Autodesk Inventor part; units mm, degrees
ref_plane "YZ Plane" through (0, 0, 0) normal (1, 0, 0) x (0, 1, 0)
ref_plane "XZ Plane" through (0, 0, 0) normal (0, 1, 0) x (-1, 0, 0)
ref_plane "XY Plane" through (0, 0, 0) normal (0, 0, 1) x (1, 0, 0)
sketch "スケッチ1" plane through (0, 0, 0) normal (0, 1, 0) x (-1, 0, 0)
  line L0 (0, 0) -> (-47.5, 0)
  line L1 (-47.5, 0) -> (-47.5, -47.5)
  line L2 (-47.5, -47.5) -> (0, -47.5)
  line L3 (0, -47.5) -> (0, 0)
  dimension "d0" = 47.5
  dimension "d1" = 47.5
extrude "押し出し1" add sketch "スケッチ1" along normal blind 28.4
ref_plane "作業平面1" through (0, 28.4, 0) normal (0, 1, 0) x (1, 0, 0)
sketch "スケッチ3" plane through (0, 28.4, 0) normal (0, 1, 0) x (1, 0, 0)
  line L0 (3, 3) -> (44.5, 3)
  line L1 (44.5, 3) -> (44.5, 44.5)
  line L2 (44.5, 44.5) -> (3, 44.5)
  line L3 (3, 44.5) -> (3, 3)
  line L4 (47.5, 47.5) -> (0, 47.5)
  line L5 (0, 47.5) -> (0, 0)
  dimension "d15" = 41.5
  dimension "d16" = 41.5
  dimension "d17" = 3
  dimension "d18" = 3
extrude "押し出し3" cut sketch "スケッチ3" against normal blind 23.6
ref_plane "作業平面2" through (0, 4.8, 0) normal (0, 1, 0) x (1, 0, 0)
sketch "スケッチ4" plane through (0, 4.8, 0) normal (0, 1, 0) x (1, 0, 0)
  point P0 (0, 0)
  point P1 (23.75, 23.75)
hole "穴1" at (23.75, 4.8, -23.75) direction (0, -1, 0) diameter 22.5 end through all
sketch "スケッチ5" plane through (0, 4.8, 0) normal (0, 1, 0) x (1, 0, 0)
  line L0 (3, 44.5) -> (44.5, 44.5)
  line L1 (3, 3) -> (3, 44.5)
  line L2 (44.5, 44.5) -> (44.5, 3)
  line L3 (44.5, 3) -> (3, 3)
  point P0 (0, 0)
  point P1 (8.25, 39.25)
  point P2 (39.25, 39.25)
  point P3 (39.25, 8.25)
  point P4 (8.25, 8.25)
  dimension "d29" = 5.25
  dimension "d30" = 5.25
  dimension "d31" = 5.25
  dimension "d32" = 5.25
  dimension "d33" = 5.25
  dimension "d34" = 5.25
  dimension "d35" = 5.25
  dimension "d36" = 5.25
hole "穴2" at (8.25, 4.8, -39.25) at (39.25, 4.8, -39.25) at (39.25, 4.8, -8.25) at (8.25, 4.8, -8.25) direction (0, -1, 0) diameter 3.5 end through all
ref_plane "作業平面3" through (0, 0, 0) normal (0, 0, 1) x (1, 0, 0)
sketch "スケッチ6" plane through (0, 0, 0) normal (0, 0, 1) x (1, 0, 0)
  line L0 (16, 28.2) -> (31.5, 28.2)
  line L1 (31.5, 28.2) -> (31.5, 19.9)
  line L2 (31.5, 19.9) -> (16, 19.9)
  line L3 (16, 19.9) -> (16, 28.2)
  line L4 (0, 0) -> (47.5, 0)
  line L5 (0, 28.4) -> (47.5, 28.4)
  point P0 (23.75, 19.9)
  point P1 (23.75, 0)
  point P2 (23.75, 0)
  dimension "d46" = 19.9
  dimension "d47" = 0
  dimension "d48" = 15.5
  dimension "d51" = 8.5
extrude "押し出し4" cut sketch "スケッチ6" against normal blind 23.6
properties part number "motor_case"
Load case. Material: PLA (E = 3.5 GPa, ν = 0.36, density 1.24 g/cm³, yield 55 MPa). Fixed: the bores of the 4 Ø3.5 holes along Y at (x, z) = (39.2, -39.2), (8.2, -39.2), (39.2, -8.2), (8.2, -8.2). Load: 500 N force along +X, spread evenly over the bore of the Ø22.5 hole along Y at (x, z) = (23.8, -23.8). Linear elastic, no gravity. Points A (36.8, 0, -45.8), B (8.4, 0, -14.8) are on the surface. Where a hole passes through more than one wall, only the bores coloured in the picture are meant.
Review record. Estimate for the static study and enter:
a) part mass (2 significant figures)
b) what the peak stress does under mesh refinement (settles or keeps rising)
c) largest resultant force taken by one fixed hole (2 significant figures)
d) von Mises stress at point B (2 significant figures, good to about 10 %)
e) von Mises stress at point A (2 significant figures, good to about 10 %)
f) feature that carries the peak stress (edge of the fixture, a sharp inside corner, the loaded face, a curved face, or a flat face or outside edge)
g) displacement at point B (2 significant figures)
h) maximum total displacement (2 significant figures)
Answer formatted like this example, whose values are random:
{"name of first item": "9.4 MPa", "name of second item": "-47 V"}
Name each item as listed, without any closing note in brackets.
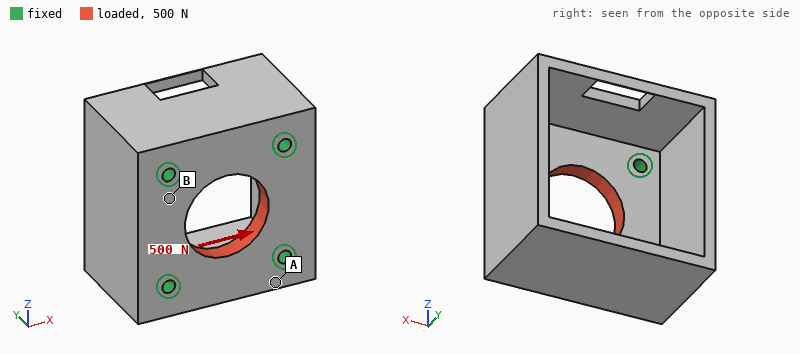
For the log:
{"part mass": "26 g", "what the peak stress does under mesh refinement": "keeps rising", "largest resultant force taken by one fixed hole": "130 N", "von Mises stress at point B": "1.6 MPa", "von Mises stress at point A": "0.45 MPa", "feature that carries the peak stress": "edge of the fixture", "displacement at point B": "7.1 µm", "maximum total displacement": "14 µm"}
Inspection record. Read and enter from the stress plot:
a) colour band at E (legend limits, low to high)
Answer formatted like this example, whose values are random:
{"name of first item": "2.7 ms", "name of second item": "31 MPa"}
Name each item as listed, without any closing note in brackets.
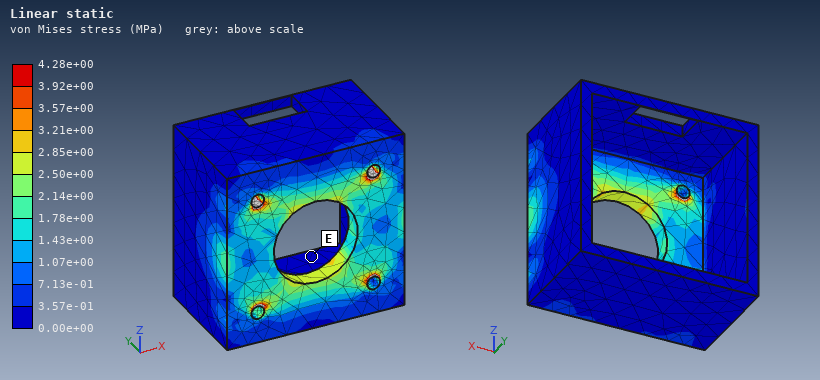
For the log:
{"colour band at E": "0.00e+00 to 3.57e-01 MPa"}
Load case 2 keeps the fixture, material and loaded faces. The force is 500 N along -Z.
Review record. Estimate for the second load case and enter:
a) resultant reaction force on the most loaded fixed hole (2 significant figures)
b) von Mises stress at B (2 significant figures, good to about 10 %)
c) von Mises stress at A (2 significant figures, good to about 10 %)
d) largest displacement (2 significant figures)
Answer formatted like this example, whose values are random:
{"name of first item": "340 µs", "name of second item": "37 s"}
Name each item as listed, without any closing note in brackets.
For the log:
{"resultant reaction force on the most loaded fixed hole": "130 N", "von Mises stress at B": "1.8 MPa", "von Mises stress at A": "0.91 MPa", "largest displacement": "15 µm"}
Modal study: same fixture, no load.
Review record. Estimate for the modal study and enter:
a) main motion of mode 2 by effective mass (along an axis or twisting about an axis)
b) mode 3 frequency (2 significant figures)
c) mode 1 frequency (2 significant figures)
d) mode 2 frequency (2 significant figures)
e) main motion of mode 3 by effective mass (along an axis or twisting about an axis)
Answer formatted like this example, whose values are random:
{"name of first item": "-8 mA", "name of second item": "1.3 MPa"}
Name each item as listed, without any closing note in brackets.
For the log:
{"main motion of mode 2 by effective mass": "along X", "mode 3 frequency": "2800 Hz", "mode 1 frequency": "2200 Hz", "mode 2 frequency": "2500 Hz", "main motion of mode 3 by effective mass": "along Z"}
